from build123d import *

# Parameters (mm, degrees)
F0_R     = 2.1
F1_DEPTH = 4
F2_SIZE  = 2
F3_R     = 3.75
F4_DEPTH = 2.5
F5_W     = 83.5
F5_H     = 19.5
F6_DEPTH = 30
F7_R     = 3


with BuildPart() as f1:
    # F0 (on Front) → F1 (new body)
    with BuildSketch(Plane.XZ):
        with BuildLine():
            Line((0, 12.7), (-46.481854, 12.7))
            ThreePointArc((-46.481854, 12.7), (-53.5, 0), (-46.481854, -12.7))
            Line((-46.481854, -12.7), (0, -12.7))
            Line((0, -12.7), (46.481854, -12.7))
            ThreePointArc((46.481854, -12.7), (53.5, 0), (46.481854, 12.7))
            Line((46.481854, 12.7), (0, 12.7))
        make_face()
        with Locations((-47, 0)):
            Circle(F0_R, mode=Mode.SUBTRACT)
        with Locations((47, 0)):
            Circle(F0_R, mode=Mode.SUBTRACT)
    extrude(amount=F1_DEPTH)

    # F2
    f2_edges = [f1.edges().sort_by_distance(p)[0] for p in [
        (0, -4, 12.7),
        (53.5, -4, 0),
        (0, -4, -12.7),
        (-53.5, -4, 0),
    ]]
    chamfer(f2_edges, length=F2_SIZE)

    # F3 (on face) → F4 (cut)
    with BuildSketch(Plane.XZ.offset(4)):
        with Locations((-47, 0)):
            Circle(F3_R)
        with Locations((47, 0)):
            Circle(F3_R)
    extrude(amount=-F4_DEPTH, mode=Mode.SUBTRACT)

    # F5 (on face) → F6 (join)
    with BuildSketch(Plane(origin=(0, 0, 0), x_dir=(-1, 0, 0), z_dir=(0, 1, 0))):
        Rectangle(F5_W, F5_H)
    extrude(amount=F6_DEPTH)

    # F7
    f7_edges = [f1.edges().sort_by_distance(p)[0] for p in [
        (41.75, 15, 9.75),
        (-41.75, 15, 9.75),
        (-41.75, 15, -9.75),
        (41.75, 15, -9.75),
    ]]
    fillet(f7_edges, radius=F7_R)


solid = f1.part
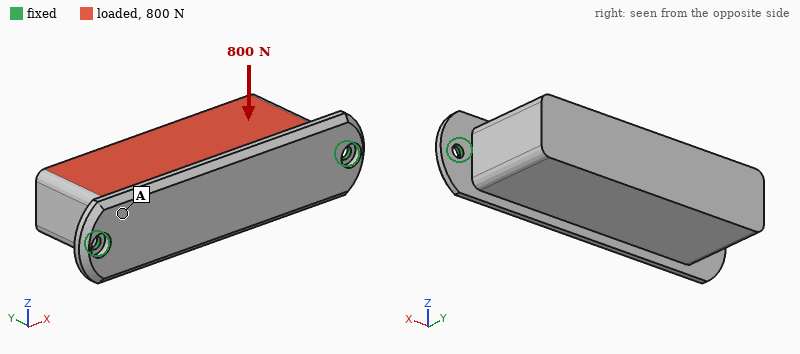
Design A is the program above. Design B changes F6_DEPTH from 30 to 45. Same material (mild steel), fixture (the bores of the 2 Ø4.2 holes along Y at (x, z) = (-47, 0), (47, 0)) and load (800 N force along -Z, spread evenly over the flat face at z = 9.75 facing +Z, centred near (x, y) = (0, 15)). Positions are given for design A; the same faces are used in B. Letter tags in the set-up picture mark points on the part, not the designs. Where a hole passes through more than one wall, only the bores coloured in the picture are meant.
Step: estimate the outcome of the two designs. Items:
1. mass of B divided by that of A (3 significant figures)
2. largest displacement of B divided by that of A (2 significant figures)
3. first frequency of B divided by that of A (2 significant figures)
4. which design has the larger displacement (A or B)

1.42
2.1
0.57
B
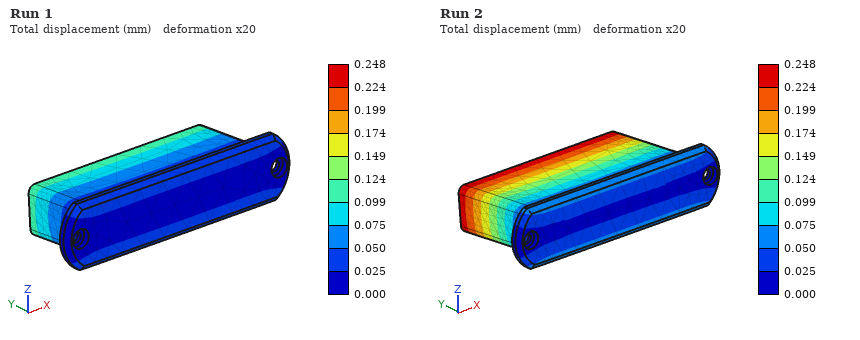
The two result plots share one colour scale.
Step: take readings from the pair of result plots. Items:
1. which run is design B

Run 2
